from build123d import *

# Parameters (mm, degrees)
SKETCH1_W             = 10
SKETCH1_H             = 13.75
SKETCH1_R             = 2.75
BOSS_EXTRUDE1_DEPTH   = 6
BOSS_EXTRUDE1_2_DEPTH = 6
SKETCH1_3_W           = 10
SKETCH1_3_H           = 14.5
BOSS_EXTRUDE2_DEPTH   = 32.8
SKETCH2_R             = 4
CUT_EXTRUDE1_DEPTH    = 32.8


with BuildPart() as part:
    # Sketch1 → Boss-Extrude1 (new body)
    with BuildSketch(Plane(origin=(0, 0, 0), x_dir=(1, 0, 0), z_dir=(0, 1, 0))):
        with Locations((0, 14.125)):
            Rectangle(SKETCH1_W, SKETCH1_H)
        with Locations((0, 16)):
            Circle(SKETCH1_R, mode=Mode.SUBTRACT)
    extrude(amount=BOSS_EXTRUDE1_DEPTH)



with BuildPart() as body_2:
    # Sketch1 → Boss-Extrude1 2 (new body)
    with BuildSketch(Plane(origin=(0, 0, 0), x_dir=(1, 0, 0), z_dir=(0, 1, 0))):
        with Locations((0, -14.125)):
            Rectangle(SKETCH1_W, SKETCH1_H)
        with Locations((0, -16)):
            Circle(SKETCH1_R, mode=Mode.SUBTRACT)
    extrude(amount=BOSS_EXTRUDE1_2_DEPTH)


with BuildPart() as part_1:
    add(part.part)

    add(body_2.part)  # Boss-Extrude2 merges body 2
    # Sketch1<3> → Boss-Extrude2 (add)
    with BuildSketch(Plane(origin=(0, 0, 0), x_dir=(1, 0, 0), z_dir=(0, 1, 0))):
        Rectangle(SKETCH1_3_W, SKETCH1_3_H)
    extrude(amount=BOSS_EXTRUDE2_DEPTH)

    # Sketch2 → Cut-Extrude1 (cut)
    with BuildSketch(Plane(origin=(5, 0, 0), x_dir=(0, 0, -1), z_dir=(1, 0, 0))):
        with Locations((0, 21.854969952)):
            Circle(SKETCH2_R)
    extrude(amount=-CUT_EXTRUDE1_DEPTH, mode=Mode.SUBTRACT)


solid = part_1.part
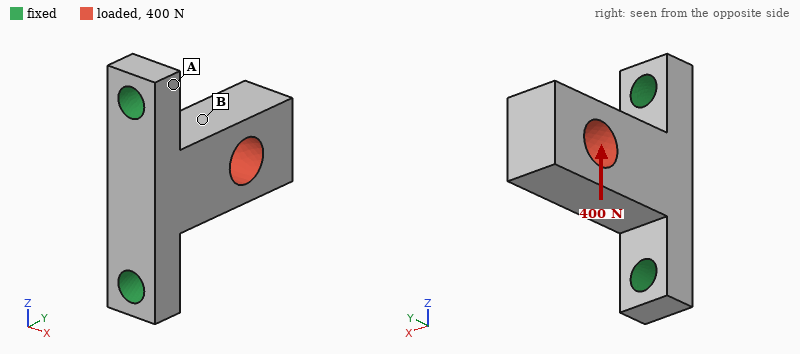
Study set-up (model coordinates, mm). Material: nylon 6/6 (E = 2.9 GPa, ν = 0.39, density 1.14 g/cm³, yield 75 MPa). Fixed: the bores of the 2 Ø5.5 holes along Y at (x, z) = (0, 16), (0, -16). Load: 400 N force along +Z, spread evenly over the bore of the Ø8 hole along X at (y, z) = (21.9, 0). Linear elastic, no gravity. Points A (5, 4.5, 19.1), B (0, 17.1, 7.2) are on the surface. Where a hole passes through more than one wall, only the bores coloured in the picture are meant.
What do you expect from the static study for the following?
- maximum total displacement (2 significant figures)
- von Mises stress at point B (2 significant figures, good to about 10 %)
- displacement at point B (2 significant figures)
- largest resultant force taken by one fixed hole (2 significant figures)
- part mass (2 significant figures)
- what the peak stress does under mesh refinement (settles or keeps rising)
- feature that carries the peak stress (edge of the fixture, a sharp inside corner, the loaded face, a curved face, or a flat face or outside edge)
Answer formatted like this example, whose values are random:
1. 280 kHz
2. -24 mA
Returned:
1. 0.55 mm
2. 11 MPa
3. 0.24 mm
4. 400 N
5. 6.4 g
6. keeps rising
7. edge of the fixture
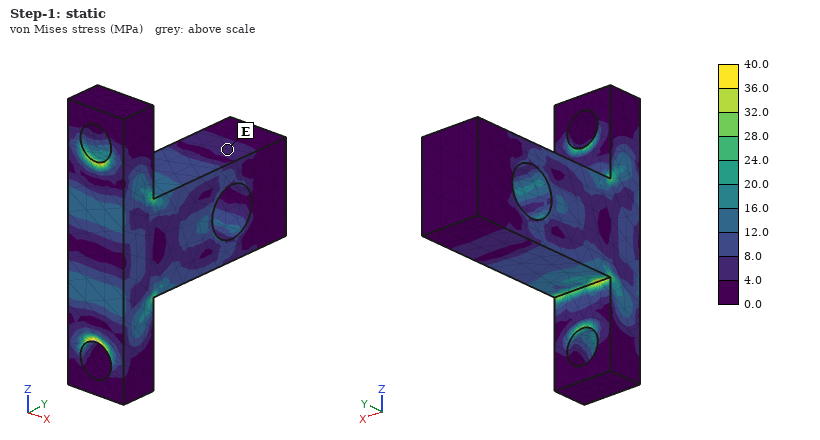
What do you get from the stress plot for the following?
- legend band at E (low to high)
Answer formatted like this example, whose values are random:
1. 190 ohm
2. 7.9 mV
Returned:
1. 4.0 to 8.0 MPa
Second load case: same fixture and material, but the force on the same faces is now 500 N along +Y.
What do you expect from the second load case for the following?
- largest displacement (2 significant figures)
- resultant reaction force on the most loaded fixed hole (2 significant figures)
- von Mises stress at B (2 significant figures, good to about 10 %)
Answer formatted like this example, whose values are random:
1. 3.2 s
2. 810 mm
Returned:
1. 0.11 mm
2. 260 N
3. 4.0 MPa
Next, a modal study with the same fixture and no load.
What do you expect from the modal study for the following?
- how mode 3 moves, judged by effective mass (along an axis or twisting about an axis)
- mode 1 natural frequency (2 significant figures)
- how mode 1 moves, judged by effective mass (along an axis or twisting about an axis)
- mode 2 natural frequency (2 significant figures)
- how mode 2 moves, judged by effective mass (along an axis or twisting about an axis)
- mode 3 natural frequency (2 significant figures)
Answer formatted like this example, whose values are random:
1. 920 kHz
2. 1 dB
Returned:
1. along Y
2. 1400 Hz
3. along X
4. 2800 Hz
5. along Z
6. 5600 Hz
